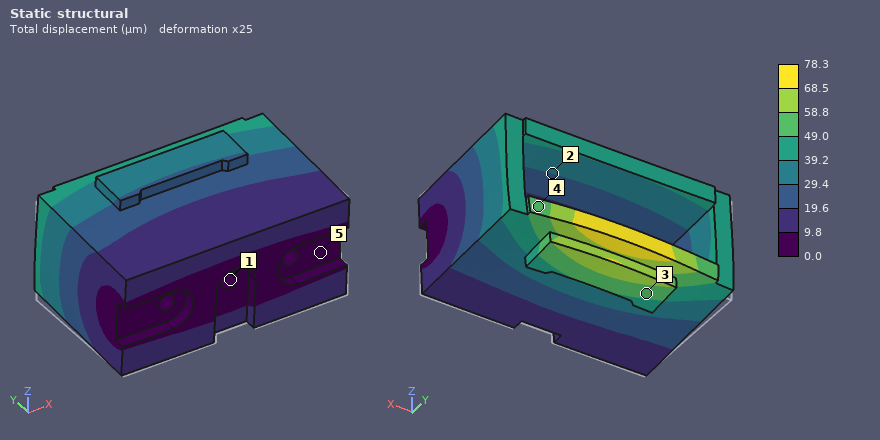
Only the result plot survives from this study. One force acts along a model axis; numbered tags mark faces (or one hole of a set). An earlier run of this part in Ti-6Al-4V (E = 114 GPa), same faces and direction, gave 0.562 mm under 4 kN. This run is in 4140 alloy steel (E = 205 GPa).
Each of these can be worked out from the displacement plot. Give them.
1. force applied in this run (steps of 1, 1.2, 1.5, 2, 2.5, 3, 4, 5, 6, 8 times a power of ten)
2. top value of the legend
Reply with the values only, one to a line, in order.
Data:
1 kN
78.3 µm
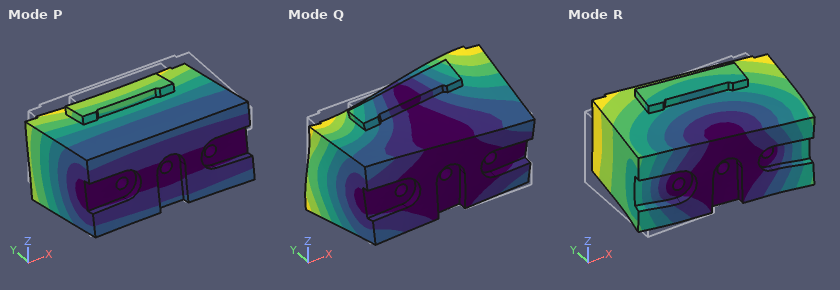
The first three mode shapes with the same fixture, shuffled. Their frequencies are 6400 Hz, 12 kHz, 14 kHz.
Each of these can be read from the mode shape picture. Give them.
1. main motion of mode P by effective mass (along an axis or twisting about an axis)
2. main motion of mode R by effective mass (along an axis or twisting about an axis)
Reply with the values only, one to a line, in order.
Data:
along Z
along X
